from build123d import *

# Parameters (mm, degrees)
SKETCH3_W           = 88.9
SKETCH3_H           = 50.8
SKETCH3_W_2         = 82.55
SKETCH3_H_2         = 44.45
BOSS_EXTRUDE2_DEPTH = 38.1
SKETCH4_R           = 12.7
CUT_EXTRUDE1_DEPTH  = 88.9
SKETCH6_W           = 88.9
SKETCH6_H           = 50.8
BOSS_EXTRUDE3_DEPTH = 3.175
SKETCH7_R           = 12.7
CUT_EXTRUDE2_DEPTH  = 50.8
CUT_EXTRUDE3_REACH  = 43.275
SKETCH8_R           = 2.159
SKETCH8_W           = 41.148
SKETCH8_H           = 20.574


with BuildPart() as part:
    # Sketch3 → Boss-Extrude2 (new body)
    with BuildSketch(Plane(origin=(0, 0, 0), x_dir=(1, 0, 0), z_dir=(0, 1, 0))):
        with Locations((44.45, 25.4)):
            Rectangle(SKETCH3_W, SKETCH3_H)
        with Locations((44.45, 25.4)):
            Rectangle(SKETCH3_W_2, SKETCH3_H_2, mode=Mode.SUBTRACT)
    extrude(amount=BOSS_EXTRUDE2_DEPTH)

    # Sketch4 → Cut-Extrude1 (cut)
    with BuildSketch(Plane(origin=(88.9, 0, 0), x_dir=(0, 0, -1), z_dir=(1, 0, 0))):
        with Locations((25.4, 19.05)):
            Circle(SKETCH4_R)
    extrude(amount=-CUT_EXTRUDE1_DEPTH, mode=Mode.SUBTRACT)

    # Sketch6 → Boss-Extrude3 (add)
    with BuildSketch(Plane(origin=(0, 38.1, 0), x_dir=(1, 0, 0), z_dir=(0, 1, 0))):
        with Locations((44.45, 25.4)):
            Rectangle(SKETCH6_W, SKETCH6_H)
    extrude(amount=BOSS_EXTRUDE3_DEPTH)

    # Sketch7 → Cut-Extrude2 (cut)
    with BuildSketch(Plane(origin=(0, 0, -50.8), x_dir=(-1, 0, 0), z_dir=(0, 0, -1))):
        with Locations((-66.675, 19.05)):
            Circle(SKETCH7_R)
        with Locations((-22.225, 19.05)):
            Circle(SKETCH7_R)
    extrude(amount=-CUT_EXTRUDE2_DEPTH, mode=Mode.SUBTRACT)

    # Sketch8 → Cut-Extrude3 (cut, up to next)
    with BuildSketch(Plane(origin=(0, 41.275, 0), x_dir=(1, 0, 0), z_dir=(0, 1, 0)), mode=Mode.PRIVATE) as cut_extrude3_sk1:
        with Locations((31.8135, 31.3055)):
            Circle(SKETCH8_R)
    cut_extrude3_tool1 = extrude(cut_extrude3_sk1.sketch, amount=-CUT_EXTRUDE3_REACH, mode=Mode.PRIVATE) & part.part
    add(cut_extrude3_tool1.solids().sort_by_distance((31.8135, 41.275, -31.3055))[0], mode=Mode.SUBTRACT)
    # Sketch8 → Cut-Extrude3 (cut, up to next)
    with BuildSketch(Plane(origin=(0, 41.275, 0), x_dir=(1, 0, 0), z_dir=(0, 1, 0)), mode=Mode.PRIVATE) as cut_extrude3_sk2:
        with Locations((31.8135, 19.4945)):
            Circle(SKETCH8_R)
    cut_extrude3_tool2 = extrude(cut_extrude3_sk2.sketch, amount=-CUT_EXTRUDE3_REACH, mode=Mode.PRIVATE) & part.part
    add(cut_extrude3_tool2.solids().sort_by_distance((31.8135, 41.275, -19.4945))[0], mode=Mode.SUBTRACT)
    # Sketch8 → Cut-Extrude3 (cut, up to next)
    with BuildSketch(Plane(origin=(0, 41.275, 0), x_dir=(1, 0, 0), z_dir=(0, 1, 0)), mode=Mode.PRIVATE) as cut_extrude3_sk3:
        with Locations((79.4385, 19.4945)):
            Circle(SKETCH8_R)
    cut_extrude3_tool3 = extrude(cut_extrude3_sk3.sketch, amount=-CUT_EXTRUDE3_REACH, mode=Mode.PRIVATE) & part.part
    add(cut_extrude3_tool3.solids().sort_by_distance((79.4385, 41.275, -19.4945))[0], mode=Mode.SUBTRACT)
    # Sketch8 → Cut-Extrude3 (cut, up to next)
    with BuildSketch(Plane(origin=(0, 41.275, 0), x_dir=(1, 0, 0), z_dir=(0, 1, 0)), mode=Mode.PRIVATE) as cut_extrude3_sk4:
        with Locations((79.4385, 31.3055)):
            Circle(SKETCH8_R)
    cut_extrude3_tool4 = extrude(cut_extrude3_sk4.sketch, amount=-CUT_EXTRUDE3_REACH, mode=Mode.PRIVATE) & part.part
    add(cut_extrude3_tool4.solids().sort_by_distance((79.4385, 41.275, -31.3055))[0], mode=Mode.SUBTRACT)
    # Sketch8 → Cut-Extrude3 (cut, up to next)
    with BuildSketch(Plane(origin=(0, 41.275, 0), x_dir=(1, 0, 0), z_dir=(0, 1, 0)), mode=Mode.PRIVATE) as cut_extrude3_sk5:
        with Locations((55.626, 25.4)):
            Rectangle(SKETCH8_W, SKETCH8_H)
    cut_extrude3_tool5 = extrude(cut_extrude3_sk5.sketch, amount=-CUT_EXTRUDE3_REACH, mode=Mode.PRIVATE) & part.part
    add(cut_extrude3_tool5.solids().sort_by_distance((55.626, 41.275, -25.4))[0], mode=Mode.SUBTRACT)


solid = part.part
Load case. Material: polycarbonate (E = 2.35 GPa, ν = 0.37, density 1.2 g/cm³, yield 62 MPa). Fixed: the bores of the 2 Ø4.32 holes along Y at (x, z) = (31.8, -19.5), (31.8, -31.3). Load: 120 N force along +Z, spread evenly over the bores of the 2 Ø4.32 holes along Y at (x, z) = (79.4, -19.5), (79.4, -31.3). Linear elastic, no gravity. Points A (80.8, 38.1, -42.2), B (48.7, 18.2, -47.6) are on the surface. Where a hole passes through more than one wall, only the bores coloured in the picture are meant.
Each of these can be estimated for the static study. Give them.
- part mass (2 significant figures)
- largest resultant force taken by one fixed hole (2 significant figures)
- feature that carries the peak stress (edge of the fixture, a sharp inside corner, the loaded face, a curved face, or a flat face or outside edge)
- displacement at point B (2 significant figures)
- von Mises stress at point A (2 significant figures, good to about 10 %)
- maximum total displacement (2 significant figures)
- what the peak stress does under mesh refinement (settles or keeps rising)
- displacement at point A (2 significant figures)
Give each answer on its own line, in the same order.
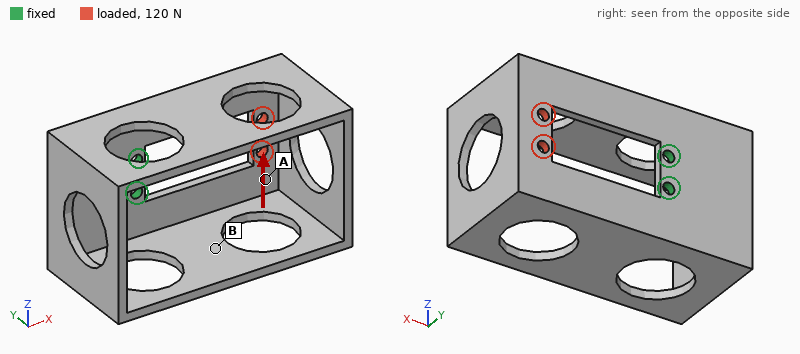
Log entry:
41 g
340 N
edge of the fixture
0.47 mm
3.5 MPa
1.2 mm
keeps rising
0.99 mm
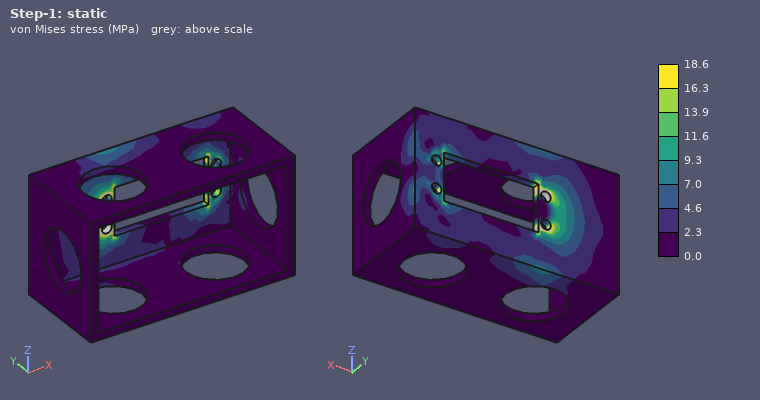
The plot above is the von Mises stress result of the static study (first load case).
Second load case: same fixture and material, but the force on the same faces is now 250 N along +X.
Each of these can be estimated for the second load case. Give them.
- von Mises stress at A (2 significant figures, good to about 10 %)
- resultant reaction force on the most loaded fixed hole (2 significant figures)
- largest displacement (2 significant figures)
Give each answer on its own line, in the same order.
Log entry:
1.8 MPa
140 N
0.18 mm
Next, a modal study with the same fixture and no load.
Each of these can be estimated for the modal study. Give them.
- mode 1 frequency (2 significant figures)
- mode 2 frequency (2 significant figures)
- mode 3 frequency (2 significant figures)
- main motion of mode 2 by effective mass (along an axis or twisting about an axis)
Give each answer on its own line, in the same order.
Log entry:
120 Hz
230 Hz
370 Hz
along Z
